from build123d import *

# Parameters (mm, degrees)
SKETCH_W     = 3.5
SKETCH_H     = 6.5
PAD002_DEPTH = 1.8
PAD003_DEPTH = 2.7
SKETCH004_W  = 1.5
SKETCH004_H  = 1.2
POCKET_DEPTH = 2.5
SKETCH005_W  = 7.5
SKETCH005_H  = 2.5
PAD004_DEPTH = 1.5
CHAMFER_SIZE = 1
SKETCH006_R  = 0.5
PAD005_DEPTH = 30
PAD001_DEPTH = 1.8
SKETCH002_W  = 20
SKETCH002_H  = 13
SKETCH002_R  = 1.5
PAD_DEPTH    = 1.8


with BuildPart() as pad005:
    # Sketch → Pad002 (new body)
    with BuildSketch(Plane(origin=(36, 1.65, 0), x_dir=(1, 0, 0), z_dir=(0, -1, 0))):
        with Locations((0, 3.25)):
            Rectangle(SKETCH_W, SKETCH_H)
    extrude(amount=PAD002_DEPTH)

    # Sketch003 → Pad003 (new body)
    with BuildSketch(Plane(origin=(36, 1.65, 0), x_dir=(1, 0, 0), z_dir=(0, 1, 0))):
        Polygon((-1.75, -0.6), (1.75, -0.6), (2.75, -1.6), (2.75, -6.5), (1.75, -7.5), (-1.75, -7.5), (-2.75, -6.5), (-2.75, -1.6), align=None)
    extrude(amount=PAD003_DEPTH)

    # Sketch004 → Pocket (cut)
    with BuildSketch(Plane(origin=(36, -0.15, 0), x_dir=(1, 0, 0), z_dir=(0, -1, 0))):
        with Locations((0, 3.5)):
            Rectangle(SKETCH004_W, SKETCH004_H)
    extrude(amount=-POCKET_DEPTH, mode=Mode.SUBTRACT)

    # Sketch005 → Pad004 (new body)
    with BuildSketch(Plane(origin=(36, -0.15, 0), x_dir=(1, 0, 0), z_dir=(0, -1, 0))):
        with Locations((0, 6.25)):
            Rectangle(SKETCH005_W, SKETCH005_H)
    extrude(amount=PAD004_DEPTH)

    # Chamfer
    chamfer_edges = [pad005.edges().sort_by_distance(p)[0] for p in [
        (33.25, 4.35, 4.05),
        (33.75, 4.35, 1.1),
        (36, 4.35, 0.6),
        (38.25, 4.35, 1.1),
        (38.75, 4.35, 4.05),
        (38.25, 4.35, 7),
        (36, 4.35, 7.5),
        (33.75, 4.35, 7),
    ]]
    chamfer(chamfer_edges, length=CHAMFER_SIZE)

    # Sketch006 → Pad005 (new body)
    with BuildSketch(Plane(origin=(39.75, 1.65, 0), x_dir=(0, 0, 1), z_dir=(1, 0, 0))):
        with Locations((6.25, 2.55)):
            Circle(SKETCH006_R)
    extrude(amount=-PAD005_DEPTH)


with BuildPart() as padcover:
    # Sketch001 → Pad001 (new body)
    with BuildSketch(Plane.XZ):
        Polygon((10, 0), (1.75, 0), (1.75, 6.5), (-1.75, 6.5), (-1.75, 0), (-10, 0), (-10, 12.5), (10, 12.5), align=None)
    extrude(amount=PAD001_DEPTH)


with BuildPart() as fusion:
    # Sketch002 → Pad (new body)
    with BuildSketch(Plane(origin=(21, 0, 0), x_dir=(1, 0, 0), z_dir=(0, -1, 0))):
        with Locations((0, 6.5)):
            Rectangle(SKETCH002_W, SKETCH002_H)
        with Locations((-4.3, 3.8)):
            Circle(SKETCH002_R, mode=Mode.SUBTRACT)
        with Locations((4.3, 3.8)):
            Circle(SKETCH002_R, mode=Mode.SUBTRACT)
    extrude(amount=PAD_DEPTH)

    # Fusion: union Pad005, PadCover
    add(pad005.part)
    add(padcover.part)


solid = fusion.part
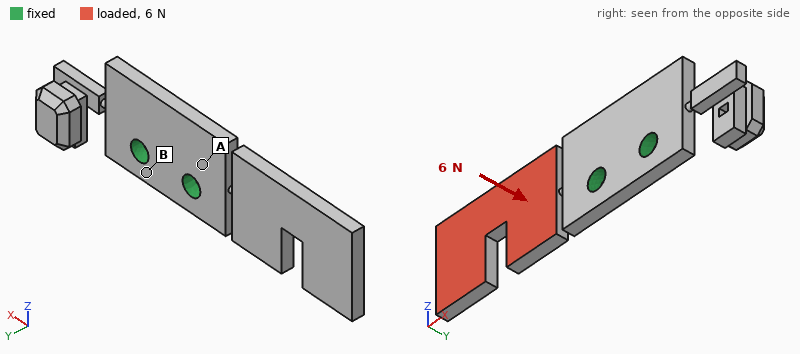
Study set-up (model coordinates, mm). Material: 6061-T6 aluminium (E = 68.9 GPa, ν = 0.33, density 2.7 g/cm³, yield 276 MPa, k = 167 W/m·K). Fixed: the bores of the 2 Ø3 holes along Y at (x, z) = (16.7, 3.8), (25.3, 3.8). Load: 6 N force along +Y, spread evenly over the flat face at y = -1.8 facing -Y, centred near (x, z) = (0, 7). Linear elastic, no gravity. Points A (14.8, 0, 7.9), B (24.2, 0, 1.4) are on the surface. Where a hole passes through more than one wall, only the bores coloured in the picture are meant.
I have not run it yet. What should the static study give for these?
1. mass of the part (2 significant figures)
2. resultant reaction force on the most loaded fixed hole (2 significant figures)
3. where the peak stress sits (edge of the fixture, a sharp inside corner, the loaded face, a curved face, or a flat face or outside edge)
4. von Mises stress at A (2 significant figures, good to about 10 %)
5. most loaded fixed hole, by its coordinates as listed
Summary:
2.7 g
8.6 N
a curved face
11 MPa
(16.7, 3.8)
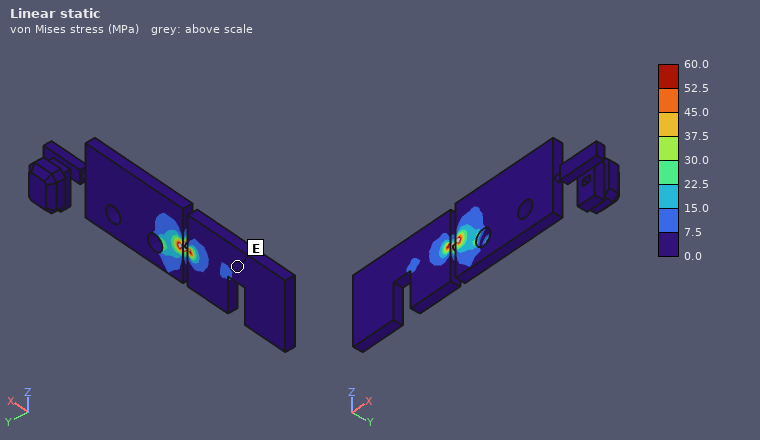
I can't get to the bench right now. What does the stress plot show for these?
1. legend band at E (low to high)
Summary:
0.0 to 7.5 MPa
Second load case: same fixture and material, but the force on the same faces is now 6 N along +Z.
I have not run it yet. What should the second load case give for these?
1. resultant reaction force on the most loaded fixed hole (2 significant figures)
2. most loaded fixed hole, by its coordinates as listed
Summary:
14 N
(16.7, 3.8)
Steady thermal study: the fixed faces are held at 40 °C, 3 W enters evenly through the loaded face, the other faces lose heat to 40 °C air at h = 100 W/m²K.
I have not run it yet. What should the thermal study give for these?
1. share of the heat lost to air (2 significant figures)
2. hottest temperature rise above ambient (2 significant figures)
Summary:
41 %
35 K
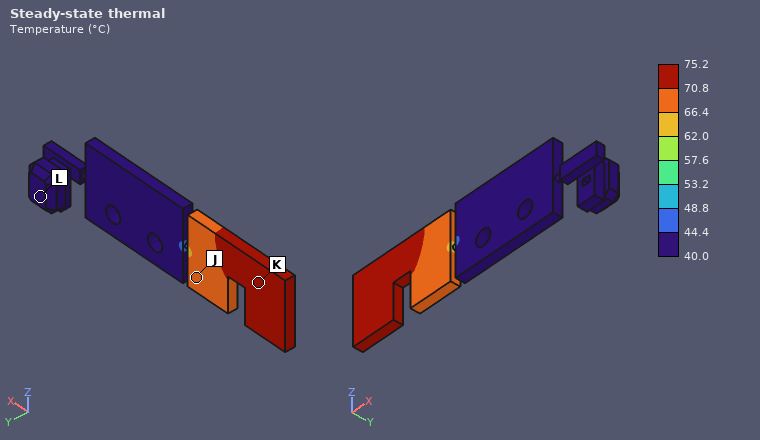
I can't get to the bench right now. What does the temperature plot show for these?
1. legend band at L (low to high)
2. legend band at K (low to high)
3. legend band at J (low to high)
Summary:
40.0 to 44.4 °C
70.8 to 75.2 °C
66.4 to 70.8 °C
